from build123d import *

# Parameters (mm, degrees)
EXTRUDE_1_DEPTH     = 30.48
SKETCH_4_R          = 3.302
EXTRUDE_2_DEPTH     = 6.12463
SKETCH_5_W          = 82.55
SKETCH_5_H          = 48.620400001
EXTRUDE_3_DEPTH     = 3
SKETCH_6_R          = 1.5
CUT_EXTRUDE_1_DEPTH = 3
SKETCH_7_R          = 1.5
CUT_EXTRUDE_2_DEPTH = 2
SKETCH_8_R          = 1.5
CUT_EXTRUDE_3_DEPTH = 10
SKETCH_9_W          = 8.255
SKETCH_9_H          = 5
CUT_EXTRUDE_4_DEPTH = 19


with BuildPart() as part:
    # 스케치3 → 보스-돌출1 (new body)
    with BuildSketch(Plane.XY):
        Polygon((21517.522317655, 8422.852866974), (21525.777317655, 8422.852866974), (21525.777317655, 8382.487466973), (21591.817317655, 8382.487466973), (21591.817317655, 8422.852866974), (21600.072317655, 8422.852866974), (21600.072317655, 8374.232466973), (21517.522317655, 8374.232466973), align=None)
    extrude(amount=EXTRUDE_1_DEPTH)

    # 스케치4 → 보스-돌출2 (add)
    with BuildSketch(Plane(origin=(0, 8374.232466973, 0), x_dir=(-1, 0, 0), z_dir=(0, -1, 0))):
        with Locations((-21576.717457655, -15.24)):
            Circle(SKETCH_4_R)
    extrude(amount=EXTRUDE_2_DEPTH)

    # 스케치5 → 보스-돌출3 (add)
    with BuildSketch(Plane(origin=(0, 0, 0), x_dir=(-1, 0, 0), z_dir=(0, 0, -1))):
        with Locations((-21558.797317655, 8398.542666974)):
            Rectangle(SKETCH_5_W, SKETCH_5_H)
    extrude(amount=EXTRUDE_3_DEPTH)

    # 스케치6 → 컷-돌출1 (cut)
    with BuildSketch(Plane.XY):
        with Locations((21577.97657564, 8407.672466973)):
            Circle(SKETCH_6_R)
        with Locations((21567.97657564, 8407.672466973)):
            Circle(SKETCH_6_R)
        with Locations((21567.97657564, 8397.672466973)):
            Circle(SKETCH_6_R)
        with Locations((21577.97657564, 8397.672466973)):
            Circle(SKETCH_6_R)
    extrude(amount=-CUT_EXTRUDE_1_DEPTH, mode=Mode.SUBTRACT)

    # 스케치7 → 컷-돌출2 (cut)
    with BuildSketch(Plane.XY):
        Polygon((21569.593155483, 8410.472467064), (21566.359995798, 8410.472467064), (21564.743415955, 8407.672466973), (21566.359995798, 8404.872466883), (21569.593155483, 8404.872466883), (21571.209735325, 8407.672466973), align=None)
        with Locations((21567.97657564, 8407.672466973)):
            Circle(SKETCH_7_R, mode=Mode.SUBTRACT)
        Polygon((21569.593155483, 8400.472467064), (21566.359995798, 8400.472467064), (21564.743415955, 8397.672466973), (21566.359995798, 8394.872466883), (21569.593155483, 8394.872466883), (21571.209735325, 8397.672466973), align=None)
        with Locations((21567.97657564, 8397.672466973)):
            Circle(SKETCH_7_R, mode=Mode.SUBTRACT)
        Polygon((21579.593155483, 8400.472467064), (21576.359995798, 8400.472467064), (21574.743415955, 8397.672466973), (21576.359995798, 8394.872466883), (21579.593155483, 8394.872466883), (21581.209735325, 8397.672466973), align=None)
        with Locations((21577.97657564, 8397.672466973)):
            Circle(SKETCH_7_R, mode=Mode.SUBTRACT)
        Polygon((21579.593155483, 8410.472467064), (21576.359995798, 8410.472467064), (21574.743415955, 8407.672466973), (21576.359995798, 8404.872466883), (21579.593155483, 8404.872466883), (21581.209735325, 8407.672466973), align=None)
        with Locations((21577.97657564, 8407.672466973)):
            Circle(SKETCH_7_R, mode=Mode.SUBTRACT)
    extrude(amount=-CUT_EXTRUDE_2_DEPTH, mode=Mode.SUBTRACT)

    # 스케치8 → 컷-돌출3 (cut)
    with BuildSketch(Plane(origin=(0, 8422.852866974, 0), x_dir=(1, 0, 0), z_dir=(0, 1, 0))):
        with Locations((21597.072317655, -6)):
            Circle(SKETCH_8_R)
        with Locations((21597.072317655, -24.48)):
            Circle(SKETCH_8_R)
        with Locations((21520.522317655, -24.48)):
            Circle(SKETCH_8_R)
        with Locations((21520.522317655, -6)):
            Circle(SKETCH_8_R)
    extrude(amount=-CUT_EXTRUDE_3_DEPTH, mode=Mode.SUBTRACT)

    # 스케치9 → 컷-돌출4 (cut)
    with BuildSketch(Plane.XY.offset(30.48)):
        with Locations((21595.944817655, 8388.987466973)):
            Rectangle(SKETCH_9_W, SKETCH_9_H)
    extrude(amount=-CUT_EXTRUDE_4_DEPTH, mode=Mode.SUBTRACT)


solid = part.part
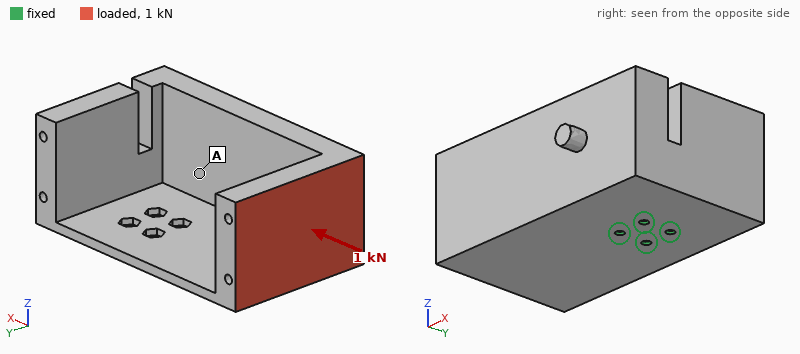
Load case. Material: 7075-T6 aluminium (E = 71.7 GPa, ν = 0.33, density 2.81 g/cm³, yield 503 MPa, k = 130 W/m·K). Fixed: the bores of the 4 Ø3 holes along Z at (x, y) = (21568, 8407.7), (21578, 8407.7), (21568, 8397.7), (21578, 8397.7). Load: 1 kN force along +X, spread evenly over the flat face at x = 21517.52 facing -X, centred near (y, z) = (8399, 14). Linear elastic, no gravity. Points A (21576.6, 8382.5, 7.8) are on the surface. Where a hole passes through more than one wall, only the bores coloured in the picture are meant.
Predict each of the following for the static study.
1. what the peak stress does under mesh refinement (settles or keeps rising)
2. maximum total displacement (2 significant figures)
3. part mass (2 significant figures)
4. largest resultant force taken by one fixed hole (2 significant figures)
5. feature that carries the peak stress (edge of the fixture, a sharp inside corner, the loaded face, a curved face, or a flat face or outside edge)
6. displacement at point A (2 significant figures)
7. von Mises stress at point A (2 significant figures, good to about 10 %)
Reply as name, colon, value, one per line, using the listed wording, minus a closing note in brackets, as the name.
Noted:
what the peak stress does under mesh refinement: keeps rising
maximum total displacement: 0.67 mm
part mass: 150 g
largest resultant force taken by one fixed hole: 1.1 kN
feature that carries the peak stress: edge of the fixture
displacement at point A: 0.11 mm
von Mises stress at point A: 20 MPa
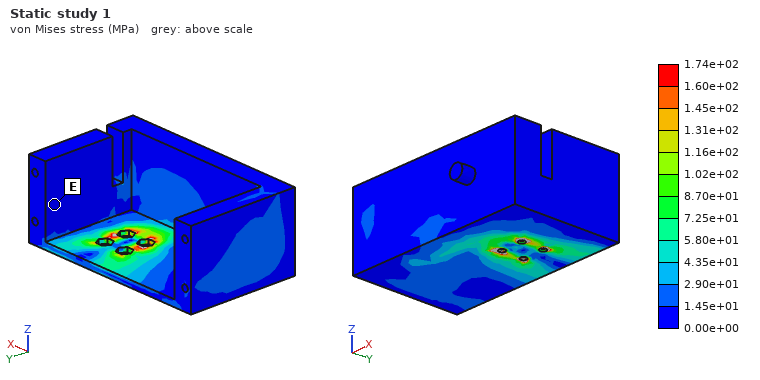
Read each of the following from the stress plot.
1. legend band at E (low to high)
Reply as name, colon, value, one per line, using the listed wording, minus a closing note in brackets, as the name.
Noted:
legend band at E: 0.00e+00 to 1.45e+01 MPa
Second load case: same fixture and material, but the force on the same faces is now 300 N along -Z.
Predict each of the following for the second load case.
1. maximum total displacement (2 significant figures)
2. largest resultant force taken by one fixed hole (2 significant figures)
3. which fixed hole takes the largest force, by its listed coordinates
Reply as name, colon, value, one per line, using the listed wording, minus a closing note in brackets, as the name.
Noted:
maximum total displacement: 0.72 mm
largest resultant force taken by one fixed hole: 1.1 kN
which fixed hole takes the largest force, by its listed coordinates: (21568, 8397.7)
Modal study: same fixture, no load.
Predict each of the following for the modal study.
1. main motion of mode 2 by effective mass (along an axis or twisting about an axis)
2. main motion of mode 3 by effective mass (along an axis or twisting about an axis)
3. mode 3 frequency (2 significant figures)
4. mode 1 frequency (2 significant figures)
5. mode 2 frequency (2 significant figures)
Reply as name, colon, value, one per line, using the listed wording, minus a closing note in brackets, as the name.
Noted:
main motion of mode 2 by effective mass: along Y
main motion of mode 3 by effective mass: along Z
mode 3 frequency: 1700 Hz
mode 1 frequency: 460 Hz
mode 2 frequency: 690 Hz
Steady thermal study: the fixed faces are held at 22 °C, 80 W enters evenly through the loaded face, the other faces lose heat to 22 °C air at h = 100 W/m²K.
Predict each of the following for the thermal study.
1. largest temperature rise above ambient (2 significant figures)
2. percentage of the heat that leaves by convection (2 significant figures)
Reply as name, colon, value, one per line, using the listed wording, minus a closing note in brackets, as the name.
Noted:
largest temperature rise above ambient: 77 K
percentage of the heat that leaves by convection: 69 %
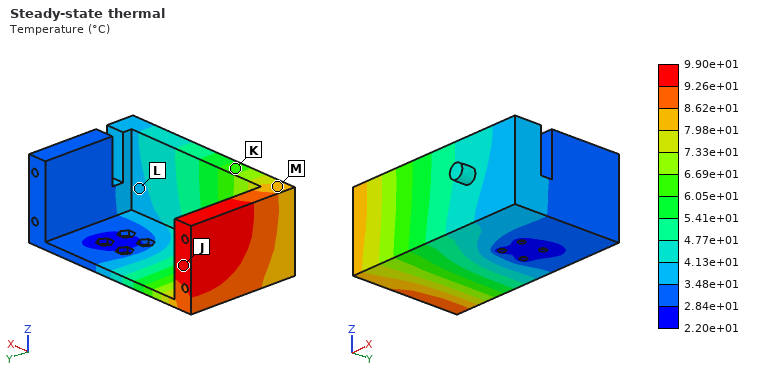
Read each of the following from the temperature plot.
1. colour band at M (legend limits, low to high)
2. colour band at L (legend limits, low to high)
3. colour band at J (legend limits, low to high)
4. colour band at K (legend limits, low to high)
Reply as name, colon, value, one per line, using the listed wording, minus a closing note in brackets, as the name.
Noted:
colour band at M: 7.98e+01 to 8.62e+01 °C
colour band at L: 3.48e+01 to 4.13e+01 °C
colour band at J: 9.26e+01 to 9.90e+01 °C
colour band at K: 6.05e+01 to 6.69e+01 °C
